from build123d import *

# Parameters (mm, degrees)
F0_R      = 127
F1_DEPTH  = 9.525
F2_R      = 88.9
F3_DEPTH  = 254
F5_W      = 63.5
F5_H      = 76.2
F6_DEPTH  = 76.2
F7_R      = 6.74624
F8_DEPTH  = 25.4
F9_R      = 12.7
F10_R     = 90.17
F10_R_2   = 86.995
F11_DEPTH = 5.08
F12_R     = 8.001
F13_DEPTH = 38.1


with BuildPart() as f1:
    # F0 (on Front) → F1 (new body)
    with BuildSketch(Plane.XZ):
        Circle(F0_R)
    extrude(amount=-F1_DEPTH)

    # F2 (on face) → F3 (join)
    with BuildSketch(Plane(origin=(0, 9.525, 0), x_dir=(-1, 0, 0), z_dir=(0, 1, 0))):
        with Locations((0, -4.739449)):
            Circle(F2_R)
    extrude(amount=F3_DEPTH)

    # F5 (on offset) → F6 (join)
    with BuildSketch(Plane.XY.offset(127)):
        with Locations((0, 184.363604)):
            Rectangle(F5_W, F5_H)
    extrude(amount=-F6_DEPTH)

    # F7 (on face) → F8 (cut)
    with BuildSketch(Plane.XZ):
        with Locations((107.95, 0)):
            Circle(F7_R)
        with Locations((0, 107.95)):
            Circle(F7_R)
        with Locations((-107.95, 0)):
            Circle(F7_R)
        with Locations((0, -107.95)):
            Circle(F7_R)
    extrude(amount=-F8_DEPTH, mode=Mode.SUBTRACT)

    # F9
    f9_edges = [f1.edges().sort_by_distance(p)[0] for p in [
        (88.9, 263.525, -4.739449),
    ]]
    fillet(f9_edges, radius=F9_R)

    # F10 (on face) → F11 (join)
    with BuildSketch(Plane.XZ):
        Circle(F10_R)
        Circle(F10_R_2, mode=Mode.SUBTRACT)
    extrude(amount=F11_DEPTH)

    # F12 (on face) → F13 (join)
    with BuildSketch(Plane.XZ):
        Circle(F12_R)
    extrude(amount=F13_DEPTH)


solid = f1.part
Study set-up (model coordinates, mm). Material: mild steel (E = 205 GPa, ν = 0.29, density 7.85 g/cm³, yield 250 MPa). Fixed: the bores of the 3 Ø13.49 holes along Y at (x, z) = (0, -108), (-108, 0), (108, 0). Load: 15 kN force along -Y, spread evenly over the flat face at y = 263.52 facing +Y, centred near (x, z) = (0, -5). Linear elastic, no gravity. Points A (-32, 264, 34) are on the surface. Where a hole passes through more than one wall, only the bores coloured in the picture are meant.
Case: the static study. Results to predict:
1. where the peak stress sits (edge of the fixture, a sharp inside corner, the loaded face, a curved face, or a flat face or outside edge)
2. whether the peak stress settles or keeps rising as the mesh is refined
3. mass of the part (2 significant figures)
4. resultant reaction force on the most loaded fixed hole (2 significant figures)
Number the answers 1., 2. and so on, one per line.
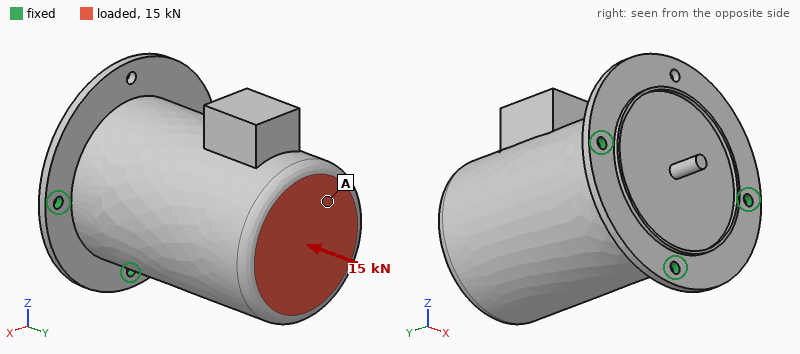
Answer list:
1. edge of the fixture
2. keeps rising
3. 55 kg
4. 7.7 kN
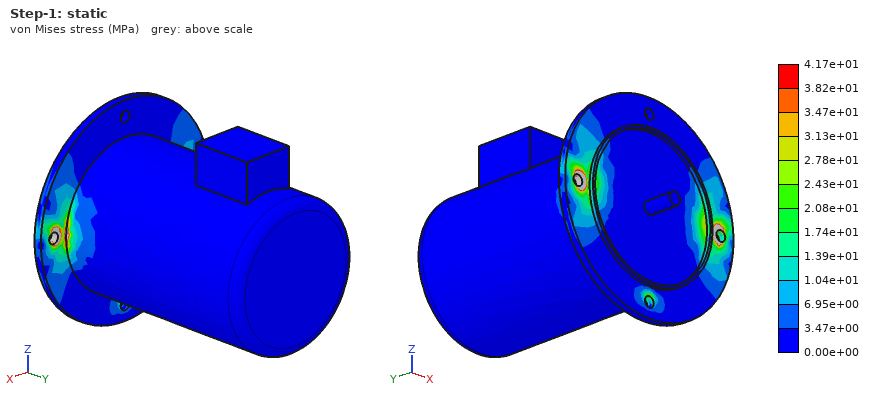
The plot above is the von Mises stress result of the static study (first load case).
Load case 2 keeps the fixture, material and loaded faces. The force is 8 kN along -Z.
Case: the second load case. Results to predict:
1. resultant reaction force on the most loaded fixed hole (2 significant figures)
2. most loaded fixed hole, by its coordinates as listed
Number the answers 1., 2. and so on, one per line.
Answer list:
1. 22 kN
2. (0, -108)
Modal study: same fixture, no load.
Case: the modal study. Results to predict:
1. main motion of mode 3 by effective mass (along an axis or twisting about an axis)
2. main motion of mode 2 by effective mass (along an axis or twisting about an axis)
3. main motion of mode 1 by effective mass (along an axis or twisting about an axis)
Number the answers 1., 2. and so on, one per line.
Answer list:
1. along Y
2. along X
3. along Z
